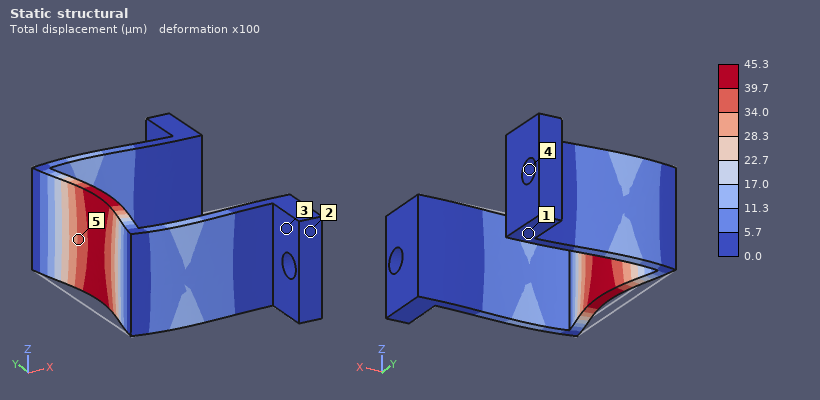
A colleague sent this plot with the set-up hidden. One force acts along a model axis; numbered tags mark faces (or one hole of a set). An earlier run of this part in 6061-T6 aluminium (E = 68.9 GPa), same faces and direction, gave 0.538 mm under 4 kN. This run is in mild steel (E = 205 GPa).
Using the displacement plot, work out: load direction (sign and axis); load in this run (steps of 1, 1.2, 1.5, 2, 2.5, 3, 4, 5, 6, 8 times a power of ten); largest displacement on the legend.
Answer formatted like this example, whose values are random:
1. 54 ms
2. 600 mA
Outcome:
1. +X
2. 1 kN
3. 45.3 µm
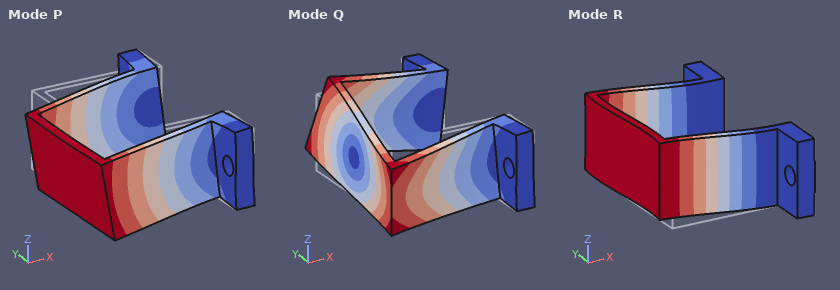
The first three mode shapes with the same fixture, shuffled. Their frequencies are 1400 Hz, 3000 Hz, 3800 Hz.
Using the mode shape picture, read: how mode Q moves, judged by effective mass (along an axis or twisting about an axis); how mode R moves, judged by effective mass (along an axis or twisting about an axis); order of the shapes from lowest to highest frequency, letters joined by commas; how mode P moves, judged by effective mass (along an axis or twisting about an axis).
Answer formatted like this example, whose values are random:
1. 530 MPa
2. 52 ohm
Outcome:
1. twisting about X
2. along Y
3. R, P, Q
4. along Z
